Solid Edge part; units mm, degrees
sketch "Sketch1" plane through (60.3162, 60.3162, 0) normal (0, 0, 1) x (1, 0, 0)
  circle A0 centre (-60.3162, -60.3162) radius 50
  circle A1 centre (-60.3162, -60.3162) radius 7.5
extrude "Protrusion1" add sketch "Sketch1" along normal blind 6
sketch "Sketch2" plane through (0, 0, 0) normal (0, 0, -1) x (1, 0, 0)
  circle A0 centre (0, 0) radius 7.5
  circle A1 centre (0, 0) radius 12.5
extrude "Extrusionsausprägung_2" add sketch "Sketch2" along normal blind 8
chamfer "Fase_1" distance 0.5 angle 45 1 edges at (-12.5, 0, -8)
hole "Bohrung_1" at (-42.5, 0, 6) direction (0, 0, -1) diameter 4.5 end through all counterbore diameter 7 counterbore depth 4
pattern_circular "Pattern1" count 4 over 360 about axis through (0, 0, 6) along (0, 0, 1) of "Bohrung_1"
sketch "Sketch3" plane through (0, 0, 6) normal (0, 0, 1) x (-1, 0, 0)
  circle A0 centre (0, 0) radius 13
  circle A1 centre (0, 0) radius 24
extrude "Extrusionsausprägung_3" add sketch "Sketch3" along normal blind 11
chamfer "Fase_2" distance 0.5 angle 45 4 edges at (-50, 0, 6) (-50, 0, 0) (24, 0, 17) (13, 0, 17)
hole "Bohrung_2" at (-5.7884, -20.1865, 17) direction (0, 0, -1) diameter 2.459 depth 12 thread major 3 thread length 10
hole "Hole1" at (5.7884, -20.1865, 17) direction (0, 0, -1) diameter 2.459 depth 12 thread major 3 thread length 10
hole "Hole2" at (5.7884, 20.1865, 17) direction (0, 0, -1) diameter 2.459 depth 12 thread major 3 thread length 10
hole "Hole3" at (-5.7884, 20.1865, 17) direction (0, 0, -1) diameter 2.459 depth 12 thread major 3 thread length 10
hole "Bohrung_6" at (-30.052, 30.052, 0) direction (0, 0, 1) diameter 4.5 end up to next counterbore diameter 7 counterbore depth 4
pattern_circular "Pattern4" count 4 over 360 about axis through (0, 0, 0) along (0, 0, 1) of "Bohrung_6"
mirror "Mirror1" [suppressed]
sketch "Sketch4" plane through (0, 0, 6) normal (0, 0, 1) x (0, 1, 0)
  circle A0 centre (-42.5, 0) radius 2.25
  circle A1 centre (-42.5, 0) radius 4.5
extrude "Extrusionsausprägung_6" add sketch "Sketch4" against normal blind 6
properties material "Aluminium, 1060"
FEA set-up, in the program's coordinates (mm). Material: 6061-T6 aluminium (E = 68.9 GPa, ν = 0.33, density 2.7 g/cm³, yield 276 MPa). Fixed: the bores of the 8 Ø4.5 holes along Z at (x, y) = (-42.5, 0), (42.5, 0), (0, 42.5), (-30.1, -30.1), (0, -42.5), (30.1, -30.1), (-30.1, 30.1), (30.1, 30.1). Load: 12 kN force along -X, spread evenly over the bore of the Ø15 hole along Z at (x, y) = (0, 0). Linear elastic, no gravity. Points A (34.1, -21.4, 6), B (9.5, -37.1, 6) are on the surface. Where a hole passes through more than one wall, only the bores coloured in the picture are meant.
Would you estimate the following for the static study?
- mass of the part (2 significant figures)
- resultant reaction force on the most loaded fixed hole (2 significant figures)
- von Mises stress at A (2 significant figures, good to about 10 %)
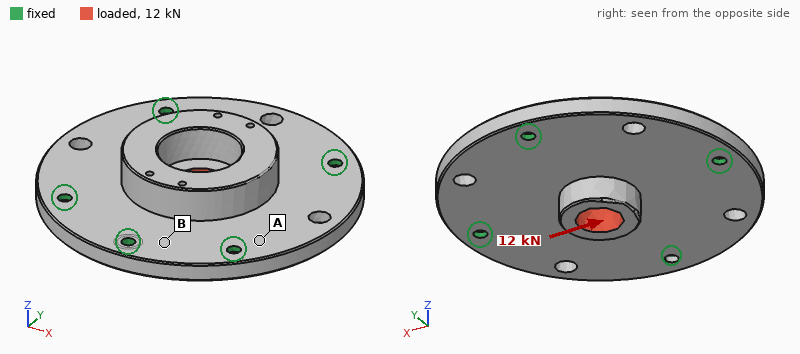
160 g
1.8 kN
19 MPa
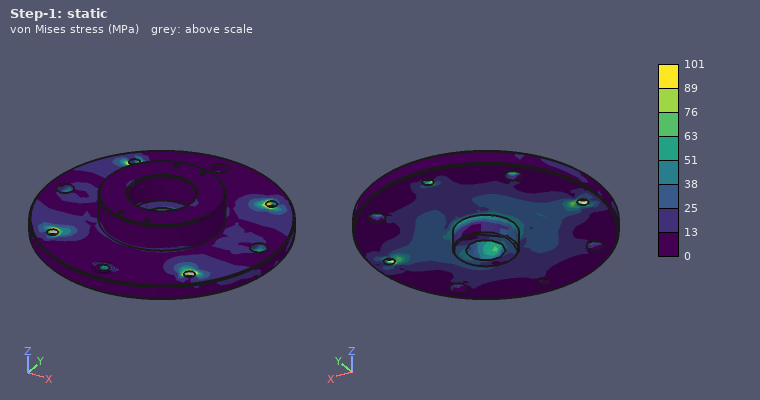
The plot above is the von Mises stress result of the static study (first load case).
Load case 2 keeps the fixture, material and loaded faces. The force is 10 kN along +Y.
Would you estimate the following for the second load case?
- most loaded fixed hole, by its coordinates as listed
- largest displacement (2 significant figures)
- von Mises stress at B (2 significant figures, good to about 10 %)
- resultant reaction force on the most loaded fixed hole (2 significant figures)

(0, -42.5)
28 µm
12 MPa
2.4 kN
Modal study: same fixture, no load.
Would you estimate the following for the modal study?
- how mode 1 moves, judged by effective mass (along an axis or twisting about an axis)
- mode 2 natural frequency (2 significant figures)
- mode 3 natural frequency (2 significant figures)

along Z
10 kHz
10 kHz
